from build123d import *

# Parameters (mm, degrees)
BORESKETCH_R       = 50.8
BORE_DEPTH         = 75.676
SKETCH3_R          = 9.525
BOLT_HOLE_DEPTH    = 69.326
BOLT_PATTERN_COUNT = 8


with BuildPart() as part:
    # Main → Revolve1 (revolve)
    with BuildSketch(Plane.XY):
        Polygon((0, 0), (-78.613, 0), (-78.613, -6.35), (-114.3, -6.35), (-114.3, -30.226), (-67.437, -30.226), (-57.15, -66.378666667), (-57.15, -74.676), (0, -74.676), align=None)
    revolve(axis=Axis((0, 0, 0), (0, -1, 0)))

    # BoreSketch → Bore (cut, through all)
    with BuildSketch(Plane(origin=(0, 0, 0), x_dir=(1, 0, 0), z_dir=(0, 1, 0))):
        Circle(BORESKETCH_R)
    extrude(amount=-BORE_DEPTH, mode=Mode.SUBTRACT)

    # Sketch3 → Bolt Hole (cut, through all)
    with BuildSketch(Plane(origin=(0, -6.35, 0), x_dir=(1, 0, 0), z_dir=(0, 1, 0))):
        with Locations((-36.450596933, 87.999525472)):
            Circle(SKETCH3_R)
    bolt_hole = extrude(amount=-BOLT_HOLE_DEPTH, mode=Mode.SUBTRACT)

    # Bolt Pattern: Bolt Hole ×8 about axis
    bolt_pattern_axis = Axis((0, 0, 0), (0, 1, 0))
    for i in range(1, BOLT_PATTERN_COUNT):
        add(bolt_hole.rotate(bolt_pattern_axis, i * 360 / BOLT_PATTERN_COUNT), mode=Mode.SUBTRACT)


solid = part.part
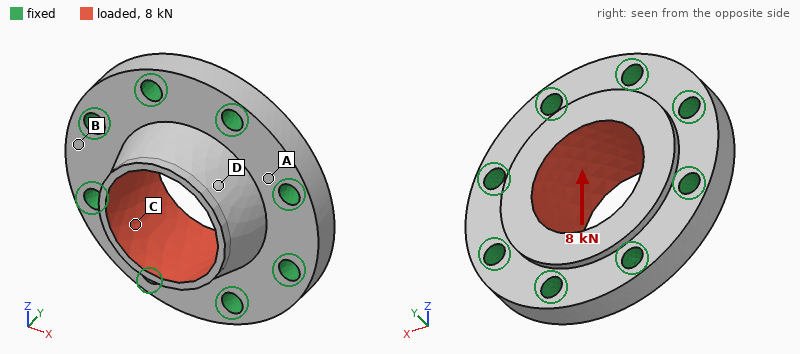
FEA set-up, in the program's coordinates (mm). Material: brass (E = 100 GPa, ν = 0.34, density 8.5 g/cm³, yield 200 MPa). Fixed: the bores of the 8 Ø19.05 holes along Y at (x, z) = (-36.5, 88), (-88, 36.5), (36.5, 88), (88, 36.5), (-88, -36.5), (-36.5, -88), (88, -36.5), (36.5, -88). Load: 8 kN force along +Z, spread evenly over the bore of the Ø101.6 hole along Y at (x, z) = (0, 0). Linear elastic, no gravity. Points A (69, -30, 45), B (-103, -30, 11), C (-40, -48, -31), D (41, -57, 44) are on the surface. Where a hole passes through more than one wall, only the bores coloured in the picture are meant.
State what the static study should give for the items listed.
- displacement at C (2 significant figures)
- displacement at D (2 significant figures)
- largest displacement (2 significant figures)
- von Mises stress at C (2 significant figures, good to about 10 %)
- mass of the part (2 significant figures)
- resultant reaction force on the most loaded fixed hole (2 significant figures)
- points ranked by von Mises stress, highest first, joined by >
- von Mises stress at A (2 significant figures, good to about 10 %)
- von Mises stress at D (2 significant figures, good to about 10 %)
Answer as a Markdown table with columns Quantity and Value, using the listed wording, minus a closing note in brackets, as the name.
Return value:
| Quantity | Value |
|---|---|
| displacement at C | 1.3 µm |
| displacement at D | 1.9 µm |
| largest displacement | 3.6 µm |
| von Mises stress at C | 2.2 MPa |
| mass of the part | 8.2 kg |
| resultant reaction force on the most loaded fixed hole | 1.4 kN |
| points ranked by von Mises stress, highest first, joined by > | C > D > A > B |
| von Mises stress at A | 0.61 MPa |
| von Mises stress at D | 1.4 MPa |
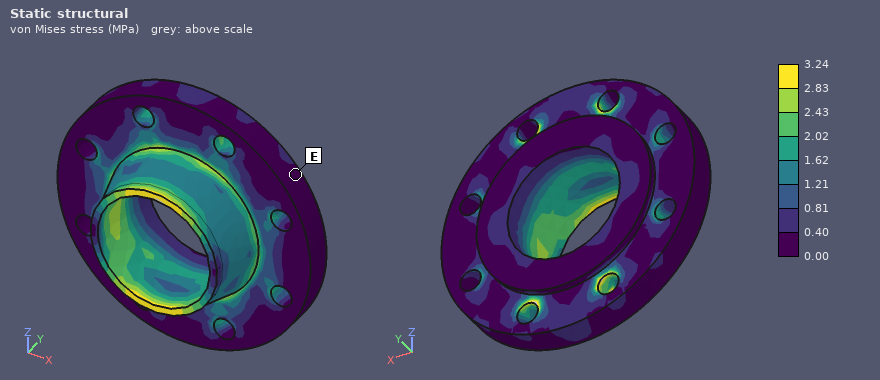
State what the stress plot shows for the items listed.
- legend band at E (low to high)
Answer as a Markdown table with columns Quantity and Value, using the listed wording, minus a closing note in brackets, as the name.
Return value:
| Quantity | Value |
|---|---|
| legend band at E | 0.00 to 0.40 MPa |
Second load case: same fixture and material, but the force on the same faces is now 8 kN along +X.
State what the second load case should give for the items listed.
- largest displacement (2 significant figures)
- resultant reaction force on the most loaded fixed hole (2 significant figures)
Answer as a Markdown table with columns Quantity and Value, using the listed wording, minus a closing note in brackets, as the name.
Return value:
| Quantity | Value |
|---|---|
| largest displacement | 3.6 µm |
| resultant reaction force on the most loaded fixed hole | 1.4 kN |
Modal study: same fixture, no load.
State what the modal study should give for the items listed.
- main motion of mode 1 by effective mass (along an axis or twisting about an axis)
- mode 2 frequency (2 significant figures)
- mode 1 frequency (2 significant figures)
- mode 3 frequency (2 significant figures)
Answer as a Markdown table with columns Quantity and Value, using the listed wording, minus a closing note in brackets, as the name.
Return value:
| Quantity | Value |
|---|---|
| main motion of mode 1 by effective mass | along Y |
| mode 2 frequency | 6400 Hz |
| mode 1 frequency | 5700 Hz |
| mode 3 frequency | 6400 Hz |
